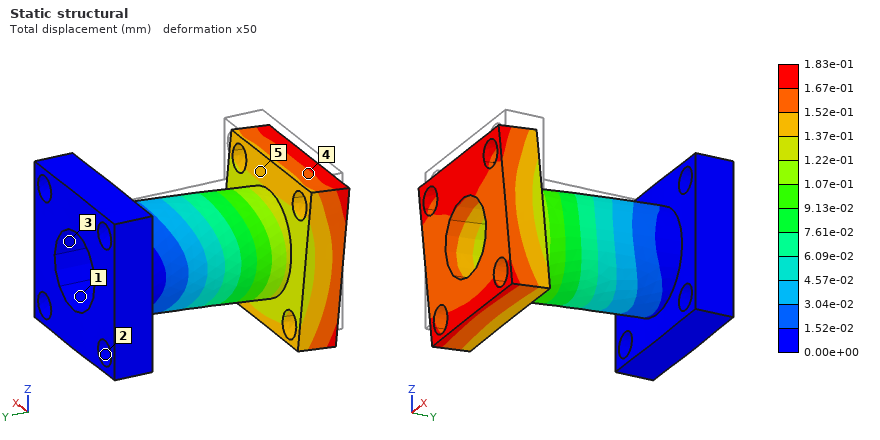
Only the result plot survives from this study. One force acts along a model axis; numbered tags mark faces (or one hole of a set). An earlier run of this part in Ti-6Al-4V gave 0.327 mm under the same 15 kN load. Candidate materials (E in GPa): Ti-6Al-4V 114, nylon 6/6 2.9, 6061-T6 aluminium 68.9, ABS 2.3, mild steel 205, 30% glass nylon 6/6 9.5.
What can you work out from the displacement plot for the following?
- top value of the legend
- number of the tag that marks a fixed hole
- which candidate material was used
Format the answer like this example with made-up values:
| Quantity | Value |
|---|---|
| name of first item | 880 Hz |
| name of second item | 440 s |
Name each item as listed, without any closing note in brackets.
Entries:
| Quantity | Value |
|---|---|
| top value of the legend | 1.83e-01 mm |
| number of the tag that marks a fixed hole | 2 |
| which candidate material was used | mild steel |
